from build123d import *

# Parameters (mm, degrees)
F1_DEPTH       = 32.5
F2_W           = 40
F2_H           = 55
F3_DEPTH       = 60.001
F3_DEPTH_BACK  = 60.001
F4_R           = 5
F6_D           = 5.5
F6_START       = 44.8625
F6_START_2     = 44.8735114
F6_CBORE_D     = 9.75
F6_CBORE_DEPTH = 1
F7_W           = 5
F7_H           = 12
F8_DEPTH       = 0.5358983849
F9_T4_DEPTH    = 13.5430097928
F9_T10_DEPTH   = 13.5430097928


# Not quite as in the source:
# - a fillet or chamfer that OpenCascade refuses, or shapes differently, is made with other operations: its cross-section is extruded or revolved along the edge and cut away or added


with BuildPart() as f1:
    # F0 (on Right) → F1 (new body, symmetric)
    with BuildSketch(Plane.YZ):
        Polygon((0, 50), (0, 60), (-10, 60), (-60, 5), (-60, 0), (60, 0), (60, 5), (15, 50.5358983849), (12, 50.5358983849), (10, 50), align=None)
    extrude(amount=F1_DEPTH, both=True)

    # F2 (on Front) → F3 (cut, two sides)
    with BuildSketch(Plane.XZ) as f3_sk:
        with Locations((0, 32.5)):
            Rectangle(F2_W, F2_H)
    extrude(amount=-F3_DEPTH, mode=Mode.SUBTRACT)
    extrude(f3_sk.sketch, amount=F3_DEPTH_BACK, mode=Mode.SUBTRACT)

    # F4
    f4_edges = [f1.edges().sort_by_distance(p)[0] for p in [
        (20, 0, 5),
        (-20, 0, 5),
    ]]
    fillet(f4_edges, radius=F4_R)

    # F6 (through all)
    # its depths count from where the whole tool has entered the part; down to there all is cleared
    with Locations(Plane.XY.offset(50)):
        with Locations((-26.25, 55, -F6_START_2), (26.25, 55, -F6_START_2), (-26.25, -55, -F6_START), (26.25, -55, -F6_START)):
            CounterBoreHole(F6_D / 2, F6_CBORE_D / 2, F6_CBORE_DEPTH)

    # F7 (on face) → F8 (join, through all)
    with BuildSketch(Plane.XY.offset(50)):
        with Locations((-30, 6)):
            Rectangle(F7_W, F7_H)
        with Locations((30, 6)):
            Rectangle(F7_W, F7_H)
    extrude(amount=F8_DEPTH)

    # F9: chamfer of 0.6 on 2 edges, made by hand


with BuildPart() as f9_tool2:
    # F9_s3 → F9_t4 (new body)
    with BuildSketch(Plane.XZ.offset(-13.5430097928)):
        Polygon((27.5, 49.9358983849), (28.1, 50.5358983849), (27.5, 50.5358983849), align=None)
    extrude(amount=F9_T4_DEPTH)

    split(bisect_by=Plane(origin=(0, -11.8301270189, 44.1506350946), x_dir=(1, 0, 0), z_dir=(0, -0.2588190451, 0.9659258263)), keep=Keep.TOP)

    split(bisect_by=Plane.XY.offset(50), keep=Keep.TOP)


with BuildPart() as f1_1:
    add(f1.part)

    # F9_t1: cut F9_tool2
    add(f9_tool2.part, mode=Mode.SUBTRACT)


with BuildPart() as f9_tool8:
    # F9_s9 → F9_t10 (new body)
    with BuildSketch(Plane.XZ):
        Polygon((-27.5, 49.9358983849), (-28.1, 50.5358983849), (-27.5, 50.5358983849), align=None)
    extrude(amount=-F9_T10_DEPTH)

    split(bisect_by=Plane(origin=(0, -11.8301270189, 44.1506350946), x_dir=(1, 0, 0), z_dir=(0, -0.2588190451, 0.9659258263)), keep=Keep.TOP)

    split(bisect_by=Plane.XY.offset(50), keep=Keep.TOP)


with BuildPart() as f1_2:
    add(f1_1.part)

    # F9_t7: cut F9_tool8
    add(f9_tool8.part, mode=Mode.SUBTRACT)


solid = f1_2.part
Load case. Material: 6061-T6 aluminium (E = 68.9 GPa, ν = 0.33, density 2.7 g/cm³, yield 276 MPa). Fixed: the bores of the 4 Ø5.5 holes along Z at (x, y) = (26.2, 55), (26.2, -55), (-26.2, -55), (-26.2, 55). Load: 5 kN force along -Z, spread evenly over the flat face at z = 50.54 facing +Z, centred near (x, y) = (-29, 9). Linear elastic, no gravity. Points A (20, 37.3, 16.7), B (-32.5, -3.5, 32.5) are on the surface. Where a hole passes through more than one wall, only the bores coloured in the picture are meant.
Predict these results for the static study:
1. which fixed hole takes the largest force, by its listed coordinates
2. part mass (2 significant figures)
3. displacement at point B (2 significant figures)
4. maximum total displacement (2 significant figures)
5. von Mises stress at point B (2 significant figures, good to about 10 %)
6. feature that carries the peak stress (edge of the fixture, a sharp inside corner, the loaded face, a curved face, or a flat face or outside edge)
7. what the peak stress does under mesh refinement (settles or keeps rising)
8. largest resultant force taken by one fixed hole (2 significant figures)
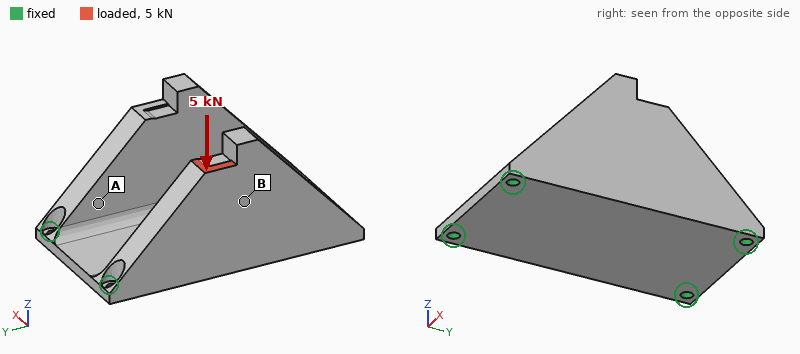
(-26.2, 55)
350 g
0.057 mm
0.10 mm
15 MPa
edge of the fixture
keeps rising
3.7 kN
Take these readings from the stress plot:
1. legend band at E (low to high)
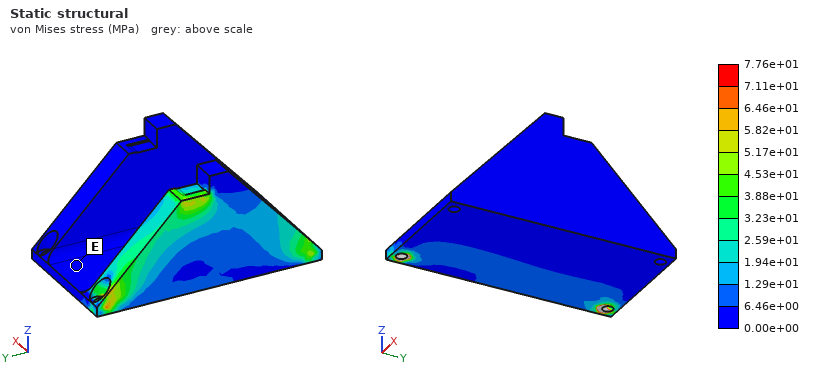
0.00e+00 to 6.46e+00 MPa
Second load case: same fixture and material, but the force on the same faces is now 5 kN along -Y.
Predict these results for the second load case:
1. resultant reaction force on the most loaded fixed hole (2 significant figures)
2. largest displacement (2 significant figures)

3.1 kN
39 µm
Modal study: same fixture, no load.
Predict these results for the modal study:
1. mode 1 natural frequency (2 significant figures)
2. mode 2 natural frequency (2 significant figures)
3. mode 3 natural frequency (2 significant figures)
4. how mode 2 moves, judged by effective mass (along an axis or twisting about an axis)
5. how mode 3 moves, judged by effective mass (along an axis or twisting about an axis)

1700 Hz
2400 Hz
5700 Hz
along X
along Z
